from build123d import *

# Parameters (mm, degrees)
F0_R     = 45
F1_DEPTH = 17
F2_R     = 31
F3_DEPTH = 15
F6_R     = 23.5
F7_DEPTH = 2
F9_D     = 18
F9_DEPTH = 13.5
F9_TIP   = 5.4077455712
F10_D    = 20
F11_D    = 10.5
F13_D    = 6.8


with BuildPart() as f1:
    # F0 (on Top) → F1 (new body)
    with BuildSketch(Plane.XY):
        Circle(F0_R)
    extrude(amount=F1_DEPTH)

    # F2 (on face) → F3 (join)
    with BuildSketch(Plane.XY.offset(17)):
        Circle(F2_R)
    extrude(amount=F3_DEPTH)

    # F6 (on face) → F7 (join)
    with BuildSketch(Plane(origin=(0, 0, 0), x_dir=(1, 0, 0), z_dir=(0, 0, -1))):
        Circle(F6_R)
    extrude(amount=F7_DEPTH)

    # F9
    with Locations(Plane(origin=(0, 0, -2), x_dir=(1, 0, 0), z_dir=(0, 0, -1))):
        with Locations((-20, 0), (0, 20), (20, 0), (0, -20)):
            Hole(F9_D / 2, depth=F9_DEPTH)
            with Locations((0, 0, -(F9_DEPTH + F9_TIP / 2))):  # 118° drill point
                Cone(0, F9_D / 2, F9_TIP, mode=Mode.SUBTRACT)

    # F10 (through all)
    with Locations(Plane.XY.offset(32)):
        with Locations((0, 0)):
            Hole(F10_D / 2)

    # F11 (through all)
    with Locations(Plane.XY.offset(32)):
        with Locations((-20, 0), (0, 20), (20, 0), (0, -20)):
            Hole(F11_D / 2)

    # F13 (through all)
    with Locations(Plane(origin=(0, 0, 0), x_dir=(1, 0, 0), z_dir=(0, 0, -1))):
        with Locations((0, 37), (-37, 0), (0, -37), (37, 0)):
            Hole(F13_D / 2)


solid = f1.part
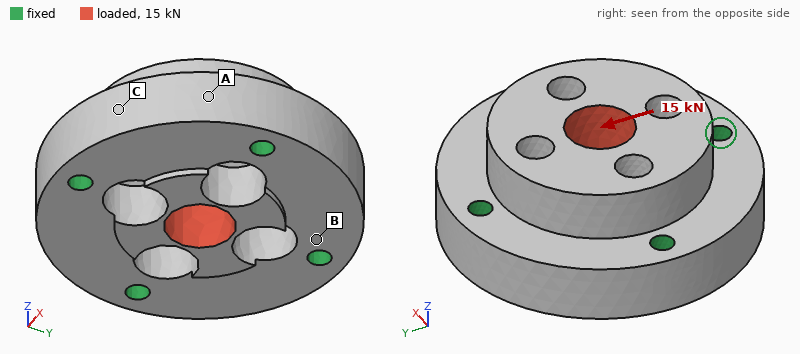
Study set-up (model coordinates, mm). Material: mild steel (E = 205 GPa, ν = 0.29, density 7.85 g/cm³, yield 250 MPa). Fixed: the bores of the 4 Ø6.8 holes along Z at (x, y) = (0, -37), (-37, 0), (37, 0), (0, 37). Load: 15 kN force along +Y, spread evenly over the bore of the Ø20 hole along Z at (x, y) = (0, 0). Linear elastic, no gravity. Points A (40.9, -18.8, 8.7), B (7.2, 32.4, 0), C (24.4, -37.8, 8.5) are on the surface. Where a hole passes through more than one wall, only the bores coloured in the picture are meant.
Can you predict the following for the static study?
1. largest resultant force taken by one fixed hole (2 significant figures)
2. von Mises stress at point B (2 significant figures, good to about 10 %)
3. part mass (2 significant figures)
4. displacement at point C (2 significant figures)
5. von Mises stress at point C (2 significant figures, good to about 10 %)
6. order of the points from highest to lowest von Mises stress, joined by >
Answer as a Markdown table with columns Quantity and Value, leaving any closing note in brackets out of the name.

| Quantity | Value |
|---|---|
| largest resultant force taken by one fixed hole | 4.3 kN |
| von Mises stress at point B | 14 MPa |
| part mass | 960 g |
| displacement at point C | 1.3 µm |
| von Mises stress at point C | 8.4 MPa |
| order of the points from highest to lowest von Mises stress, joined by > | B > C > A |
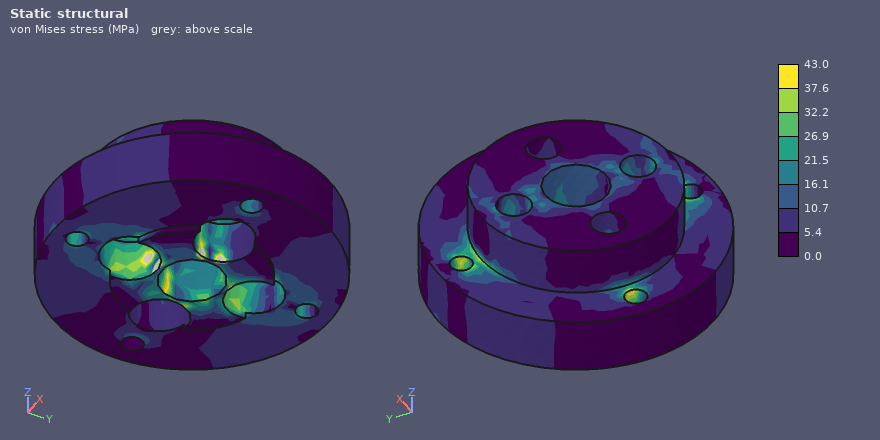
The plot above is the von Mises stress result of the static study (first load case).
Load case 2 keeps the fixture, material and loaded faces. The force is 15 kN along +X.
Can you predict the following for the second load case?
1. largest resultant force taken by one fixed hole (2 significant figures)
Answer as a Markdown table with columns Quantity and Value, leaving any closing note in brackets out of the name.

| Quantity | Value |
|---|---|
| largest resultant force taken by one fixed hole | 4.3 kN |
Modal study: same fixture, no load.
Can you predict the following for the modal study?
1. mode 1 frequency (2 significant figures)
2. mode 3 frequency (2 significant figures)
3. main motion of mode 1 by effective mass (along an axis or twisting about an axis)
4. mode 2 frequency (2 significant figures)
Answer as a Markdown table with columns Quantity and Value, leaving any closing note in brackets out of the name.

| Quantity | Value |
|---|---|
| mode 1 frequency | 16 kHz |
| mode 3 frequency | 17 kHz |
| main motion of mode 1 by effective mass | along Z |
| mode 2 frequency | 17 kHz |
